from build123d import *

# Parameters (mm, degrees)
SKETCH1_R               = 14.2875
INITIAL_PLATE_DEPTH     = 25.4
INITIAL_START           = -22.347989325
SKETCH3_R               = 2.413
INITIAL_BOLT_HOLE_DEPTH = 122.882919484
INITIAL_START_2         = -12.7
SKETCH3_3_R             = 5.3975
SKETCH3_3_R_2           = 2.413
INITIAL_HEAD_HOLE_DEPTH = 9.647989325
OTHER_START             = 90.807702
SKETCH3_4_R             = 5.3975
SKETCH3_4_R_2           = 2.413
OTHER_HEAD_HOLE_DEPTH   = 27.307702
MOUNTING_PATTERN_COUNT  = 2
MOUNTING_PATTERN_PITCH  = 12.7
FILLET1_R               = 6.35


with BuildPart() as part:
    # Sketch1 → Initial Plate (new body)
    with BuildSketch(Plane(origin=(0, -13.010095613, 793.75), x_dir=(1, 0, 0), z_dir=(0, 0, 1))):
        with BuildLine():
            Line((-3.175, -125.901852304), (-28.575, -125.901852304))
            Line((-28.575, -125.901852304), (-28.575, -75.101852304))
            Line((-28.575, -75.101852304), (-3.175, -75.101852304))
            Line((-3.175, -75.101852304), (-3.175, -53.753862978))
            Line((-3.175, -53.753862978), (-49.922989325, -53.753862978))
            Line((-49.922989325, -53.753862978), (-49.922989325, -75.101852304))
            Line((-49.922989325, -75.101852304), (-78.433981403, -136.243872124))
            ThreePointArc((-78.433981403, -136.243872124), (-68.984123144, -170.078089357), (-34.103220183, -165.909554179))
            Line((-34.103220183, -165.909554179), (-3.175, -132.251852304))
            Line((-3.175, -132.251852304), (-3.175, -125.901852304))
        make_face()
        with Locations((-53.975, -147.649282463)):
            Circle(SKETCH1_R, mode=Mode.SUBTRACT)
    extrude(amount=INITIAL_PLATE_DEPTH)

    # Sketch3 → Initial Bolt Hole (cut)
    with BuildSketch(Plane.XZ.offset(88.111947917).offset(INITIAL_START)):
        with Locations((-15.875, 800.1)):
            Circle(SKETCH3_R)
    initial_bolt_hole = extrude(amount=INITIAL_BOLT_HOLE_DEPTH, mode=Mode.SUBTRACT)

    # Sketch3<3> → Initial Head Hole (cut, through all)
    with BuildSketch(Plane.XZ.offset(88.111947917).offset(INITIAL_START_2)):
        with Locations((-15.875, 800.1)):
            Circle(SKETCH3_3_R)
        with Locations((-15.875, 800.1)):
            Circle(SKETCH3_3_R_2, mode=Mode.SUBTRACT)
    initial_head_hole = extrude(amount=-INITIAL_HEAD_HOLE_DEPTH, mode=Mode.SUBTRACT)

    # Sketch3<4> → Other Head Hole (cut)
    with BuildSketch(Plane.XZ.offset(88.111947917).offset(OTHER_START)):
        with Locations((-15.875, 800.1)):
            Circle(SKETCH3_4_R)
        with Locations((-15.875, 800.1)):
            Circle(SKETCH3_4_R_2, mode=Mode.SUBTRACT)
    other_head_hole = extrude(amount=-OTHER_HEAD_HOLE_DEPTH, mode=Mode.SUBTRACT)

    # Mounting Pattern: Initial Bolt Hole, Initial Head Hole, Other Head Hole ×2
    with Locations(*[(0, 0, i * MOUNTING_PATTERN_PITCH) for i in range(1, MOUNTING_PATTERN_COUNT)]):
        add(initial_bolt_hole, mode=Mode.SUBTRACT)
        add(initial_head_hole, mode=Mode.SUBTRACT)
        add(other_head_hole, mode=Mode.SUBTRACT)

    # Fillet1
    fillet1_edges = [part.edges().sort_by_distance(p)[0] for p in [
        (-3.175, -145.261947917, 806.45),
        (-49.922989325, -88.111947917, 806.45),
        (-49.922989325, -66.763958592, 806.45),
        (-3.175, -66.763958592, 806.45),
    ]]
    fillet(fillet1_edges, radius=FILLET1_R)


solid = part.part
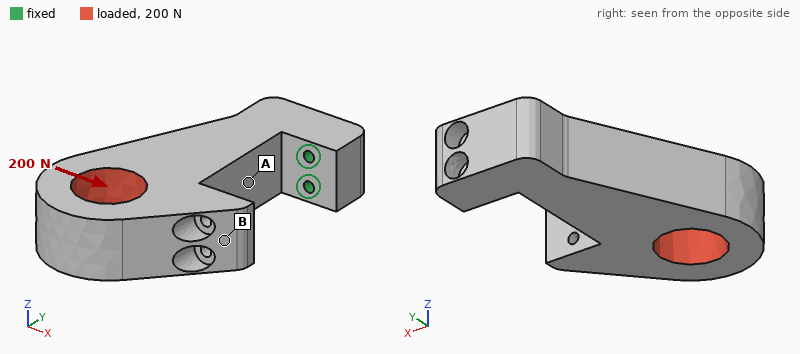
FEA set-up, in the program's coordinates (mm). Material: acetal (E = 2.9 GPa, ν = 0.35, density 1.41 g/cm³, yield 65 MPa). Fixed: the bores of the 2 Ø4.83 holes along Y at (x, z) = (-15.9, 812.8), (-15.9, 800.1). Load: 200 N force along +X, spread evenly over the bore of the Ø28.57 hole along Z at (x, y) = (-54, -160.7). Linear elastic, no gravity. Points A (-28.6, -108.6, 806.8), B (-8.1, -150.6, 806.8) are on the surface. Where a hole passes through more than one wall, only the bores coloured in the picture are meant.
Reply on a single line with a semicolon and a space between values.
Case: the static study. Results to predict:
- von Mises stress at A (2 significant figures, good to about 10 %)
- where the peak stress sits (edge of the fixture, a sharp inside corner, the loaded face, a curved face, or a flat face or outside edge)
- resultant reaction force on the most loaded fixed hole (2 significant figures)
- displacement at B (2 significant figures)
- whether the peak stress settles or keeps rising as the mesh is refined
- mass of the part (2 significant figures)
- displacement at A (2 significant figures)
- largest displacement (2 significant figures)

2.9 MPa; edge of the fixture; 130 N; 1.1 mm; keeps rising; 160 g; 0.38 mm; 1.7 mm
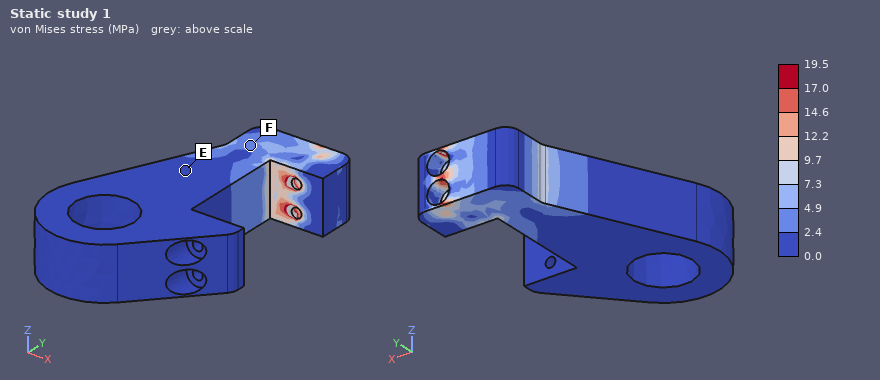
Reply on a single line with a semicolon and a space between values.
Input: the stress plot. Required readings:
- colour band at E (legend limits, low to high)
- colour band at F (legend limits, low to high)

0.0 to 2.4 MPa; 2.4 to 4.9 MPa
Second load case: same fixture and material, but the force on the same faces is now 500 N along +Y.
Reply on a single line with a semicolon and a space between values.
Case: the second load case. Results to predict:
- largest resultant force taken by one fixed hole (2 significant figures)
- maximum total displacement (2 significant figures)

260 N; 1.5 mm
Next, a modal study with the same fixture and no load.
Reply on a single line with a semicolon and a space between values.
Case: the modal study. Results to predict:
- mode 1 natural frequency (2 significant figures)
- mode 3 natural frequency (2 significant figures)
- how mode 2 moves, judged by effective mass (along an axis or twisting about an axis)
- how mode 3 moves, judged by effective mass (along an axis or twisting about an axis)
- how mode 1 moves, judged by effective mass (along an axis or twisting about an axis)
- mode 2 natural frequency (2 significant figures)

200 Hz; 760 Hz; along Z; twisting about Y; along X; 230 Hz
